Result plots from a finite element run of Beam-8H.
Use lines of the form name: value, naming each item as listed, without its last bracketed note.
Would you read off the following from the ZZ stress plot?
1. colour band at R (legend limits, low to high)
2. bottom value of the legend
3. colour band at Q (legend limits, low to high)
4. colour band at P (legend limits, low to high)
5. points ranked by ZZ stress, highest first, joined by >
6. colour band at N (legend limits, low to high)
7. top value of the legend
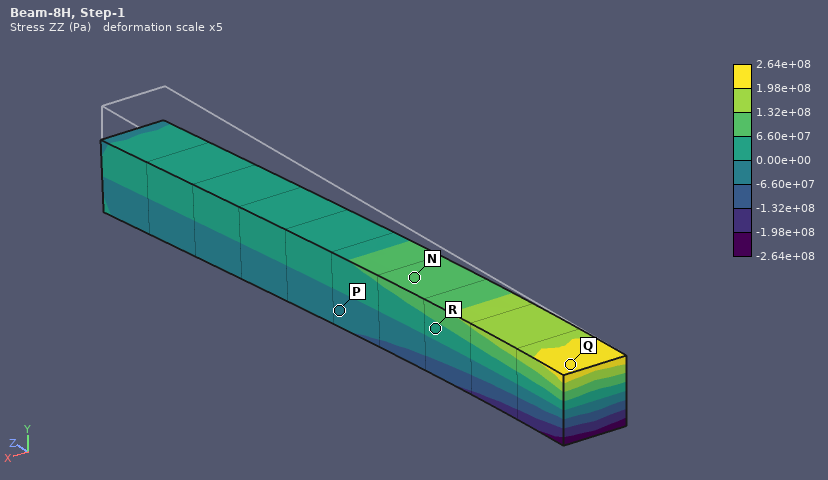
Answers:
colour band at R: 0.00e+00 to 6.60e+07 Pa
bottom value of the legend: -2.64e+08 Pa
colour band at Q: 1.98e+08 to 2.64e+08 Pa
colour band at P: -6.60e+07 to 0.00e+00 Pa
points ranked by ZZ stress, highest first, joined by >: Q > N > R > P
colour band at N: 6.60e+07 to 1.32e+08 Pa
top value of the legend: 2.64e+08 Pa
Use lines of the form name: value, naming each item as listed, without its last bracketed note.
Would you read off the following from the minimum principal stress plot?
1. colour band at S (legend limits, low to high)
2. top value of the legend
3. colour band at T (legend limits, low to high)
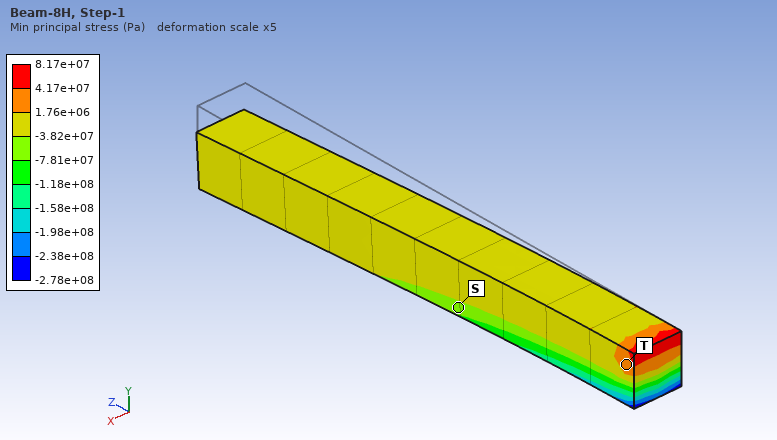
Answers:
colour band at S: -7.81e+07 to -3.82e+07 Pa
top value of the legend: 8.17e+07 Pa
colour band at T: 1.76e+06 to 4.17e+07 Pa
